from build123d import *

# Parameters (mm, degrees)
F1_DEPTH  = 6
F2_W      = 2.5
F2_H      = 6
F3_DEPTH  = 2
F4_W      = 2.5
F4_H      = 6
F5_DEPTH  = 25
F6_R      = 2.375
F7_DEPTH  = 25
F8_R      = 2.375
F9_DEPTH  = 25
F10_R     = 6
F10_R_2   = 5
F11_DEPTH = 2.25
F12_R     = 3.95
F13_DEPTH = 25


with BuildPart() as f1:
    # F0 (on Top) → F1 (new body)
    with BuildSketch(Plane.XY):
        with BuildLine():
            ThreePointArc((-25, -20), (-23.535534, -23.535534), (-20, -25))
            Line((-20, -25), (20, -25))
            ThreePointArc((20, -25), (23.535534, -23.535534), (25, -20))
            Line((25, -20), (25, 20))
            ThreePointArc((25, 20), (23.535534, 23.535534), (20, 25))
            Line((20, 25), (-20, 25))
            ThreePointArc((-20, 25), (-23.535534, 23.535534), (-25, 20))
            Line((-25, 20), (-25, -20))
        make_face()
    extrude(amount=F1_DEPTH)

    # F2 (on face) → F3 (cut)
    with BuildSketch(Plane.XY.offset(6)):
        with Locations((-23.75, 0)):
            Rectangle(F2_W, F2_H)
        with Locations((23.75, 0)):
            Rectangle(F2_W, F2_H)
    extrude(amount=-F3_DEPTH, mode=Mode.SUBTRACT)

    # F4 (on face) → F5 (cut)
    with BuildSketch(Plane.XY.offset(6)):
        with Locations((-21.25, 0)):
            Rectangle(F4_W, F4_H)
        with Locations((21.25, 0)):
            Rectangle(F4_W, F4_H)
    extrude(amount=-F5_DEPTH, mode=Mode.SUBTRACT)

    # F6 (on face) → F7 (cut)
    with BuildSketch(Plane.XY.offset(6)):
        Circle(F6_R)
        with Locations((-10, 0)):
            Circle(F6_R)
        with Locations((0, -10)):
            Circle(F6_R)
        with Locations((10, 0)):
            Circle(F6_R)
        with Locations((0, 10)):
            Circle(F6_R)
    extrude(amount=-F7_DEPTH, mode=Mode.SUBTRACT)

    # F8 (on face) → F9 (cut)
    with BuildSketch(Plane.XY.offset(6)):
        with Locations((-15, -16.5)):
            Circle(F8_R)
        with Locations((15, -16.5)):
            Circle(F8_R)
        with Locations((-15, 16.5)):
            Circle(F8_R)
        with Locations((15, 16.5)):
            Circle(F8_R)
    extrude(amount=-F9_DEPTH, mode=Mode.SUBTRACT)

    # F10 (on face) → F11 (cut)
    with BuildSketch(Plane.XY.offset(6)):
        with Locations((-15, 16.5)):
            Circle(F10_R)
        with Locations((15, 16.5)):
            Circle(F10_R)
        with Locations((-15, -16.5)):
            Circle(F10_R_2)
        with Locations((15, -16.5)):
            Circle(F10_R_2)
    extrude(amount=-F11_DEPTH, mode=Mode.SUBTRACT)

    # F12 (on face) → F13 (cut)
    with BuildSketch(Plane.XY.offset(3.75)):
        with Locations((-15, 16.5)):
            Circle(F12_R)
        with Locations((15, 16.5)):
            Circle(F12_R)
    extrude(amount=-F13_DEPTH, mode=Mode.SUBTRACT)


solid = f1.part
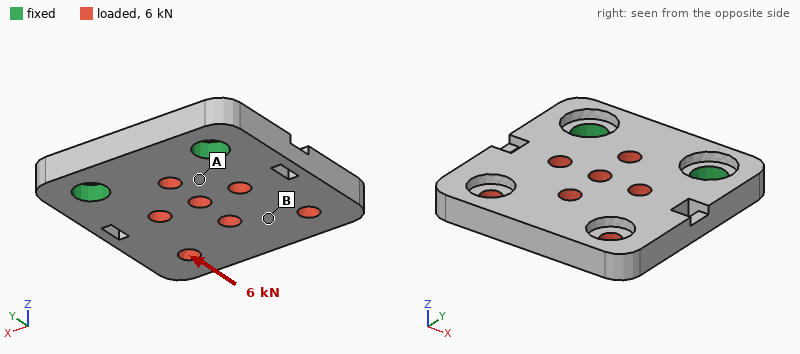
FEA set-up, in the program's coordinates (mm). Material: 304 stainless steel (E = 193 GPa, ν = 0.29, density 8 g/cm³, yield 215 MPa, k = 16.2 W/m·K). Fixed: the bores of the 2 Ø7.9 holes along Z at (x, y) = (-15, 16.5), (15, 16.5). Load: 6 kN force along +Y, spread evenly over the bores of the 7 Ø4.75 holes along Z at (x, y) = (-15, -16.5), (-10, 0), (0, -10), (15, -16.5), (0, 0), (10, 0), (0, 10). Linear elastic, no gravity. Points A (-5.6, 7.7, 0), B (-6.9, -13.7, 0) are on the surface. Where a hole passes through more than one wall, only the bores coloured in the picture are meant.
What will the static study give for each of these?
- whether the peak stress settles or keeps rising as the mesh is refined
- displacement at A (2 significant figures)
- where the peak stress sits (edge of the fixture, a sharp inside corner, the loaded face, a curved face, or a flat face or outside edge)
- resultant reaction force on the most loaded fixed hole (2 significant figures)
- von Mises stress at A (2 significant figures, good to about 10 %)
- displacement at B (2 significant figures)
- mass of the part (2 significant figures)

keeps rising
2.5 µm
edge of the fixture
3.1 kN
27 MPa
5.8 µm
100 g
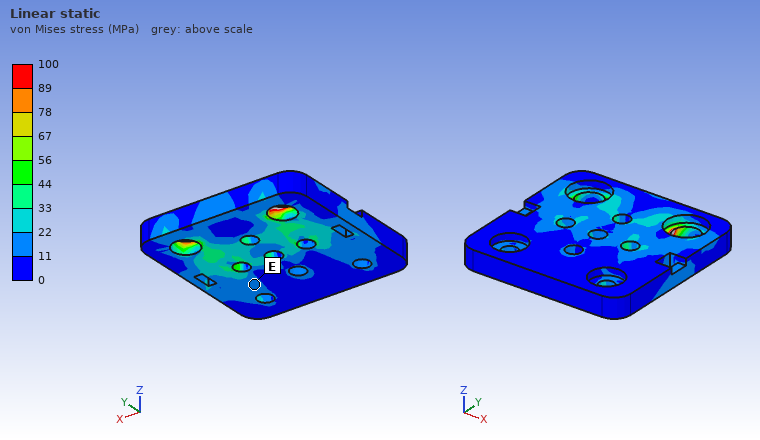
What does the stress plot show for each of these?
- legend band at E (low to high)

11 to 22 MPa
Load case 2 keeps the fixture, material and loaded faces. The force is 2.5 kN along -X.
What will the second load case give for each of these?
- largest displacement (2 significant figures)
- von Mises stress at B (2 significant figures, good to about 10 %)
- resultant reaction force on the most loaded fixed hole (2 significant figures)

7.2 µm
5.9 MPa
1.8 kN
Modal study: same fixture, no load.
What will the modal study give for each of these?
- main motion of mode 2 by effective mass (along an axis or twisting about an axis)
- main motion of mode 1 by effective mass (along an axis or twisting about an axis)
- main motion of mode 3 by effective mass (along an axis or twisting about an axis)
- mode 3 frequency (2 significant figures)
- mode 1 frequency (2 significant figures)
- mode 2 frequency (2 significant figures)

twisting about Y
along Z
along X
12 kHz
2400 Hz
5300 Hz
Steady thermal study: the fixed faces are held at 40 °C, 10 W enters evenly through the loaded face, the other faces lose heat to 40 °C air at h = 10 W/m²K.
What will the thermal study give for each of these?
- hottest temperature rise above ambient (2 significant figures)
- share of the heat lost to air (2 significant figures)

45 K
16 %
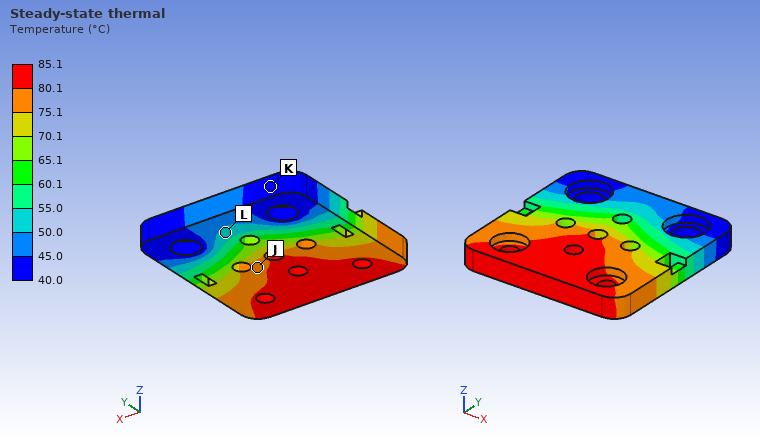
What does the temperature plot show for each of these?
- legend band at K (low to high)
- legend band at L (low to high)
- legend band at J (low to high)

40.0 to 45.0 °C
50.0 to 55.0 °C
75.1 to 80.1 °C
